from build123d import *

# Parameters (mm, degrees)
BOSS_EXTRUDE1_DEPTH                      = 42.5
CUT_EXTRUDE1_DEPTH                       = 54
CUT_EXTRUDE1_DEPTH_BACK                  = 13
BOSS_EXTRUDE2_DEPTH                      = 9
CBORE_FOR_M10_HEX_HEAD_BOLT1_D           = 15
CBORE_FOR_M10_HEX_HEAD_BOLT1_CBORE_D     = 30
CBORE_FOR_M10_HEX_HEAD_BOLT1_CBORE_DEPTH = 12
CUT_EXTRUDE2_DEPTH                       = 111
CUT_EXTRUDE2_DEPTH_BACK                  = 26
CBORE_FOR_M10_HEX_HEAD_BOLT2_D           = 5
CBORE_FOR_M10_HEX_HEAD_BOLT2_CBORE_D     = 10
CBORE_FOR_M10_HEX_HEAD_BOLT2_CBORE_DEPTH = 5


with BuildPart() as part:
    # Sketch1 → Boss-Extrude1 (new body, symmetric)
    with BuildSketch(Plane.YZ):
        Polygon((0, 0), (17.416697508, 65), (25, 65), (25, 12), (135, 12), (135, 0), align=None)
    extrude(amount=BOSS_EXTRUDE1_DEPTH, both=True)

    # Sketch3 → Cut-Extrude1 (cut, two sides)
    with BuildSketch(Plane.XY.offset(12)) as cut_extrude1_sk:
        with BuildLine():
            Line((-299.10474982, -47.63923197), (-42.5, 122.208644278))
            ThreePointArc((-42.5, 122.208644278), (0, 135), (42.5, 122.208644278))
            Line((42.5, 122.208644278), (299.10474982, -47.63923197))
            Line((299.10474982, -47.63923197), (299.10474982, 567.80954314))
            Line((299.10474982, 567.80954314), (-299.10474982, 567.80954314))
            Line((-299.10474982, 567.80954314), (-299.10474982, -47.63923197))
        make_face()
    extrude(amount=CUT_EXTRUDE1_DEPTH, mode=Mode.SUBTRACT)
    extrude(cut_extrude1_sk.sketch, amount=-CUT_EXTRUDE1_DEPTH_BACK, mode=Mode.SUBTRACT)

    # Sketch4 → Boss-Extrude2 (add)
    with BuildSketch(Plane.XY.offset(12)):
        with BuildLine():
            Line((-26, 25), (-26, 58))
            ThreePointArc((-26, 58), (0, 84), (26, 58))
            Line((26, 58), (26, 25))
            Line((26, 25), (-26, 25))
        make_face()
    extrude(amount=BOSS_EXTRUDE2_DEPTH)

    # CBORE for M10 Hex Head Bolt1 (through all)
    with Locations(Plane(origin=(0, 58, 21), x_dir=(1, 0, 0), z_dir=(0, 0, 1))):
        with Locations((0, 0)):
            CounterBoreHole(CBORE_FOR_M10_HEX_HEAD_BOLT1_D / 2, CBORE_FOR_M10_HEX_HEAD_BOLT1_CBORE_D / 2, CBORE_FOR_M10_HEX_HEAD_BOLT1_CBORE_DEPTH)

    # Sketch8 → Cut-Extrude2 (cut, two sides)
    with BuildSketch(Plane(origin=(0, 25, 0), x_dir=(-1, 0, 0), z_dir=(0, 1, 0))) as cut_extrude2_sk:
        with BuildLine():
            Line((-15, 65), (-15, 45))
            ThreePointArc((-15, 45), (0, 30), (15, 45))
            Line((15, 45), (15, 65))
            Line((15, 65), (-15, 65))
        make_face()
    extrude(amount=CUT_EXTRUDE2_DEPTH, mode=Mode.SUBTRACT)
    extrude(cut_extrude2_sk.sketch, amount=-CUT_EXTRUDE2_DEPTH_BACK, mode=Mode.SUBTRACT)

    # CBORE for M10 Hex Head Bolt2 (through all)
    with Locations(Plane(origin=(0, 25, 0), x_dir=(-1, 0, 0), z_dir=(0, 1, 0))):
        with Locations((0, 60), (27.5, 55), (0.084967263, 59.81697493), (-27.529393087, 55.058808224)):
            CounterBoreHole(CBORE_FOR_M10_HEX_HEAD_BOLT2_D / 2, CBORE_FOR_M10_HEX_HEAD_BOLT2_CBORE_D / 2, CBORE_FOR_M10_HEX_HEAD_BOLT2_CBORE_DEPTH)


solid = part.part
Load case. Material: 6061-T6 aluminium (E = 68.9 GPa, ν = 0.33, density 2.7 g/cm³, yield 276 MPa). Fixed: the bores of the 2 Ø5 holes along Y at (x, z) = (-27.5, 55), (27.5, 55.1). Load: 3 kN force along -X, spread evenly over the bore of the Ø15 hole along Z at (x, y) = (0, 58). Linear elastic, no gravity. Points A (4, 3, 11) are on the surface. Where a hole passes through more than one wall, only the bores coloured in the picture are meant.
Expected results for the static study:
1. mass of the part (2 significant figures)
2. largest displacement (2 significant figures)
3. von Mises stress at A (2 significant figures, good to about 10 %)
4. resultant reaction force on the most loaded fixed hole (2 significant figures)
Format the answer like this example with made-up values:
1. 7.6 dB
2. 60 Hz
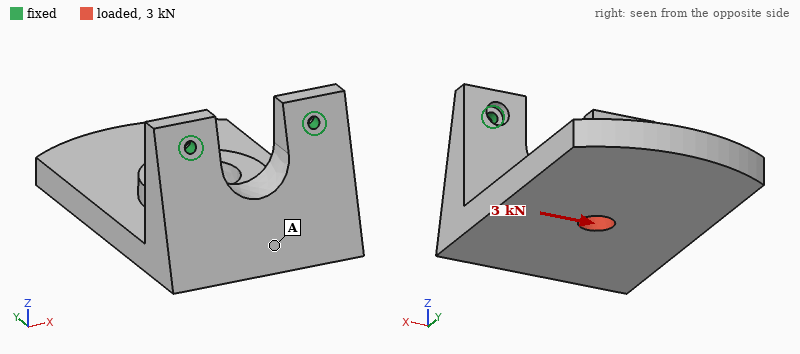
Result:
1. 540 g
2. 0.26 mm
3. 14 MPa
4. 3.5 kN
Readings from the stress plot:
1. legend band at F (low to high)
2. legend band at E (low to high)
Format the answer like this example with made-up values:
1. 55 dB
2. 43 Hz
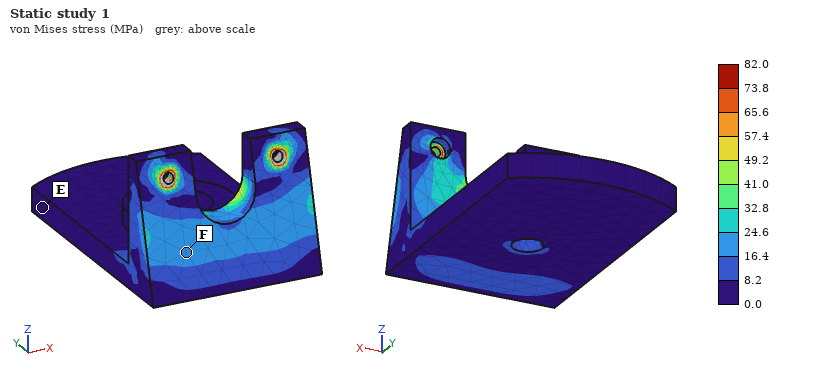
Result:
1. 16.4 to 24.6 MPa
2. 0.0 to 8.2 MPa
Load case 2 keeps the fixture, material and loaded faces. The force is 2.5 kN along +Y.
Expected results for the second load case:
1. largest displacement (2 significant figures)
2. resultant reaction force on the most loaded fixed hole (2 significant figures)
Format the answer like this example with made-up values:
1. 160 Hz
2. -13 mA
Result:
1. 1.4 mm
2. 1.3 kN
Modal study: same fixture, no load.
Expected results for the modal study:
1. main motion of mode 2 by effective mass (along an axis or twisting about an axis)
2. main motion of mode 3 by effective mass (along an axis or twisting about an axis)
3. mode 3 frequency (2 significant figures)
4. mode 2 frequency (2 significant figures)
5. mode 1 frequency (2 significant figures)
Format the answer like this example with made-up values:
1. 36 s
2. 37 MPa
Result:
1. along X
2. along Y
3. 1700 Hz
4. 920 Hz
5. 340 Hz
